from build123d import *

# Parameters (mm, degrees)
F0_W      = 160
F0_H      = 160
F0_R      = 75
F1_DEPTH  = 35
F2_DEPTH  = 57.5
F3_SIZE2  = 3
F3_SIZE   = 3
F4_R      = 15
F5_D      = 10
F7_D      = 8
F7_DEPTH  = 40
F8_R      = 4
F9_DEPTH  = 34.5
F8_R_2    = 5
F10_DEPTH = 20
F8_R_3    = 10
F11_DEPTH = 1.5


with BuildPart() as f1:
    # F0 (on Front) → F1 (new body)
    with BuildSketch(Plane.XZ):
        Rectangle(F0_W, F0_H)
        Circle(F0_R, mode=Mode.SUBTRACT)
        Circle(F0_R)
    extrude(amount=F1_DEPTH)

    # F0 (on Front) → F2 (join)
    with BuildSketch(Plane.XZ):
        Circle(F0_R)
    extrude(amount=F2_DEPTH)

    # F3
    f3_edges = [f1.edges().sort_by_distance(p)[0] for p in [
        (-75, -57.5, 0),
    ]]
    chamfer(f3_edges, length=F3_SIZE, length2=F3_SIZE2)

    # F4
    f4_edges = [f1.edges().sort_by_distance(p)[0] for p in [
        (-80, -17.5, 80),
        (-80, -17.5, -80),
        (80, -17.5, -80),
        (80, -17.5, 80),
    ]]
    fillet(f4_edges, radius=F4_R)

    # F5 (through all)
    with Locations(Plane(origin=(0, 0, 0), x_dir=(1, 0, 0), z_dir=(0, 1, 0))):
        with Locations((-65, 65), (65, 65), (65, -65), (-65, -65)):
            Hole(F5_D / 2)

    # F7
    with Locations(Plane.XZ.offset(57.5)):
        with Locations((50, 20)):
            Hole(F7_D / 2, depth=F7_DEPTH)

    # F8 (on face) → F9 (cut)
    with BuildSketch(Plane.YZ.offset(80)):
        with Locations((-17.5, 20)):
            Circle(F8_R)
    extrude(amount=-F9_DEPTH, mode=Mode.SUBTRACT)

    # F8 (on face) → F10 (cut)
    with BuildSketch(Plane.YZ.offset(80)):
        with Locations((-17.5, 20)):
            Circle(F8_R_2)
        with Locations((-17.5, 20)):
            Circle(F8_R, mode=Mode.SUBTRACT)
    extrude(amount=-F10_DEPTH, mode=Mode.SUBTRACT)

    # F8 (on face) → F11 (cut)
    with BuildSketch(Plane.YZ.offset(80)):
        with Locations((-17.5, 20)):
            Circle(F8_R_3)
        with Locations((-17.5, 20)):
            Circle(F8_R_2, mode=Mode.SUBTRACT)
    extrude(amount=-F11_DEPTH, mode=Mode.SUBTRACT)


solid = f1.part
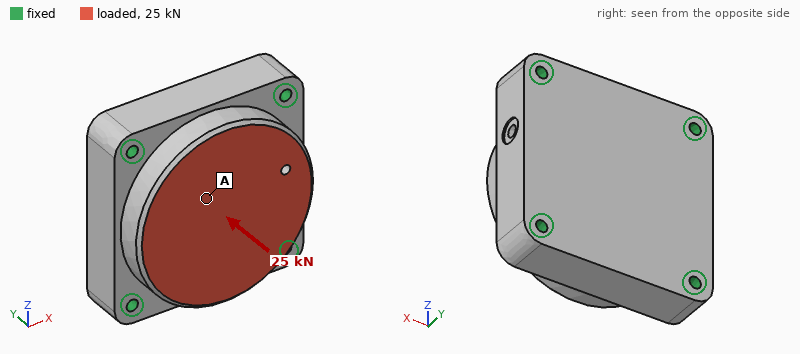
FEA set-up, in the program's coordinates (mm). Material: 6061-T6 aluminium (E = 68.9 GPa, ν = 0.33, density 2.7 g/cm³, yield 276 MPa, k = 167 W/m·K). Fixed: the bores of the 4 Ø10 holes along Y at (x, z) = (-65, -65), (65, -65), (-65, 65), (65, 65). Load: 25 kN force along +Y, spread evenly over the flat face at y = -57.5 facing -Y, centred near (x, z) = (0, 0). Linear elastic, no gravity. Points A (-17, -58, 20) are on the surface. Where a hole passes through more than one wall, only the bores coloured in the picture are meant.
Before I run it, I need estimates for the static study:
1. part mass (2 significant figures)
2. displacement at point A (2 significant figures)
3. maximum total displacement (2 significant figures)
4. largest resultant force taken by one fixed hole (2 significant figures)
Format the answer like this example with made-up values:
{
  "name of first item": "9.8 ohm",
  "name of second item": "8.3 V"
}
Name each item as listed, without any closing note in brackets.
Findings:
{
  "part mass": "3.4 kg",
  "displacement at point A": "9.3 µm",
  "maximum total displacement": "9.8 µm",
  "largest resultant force taken by one fixed hole": "6.6 kN"
}
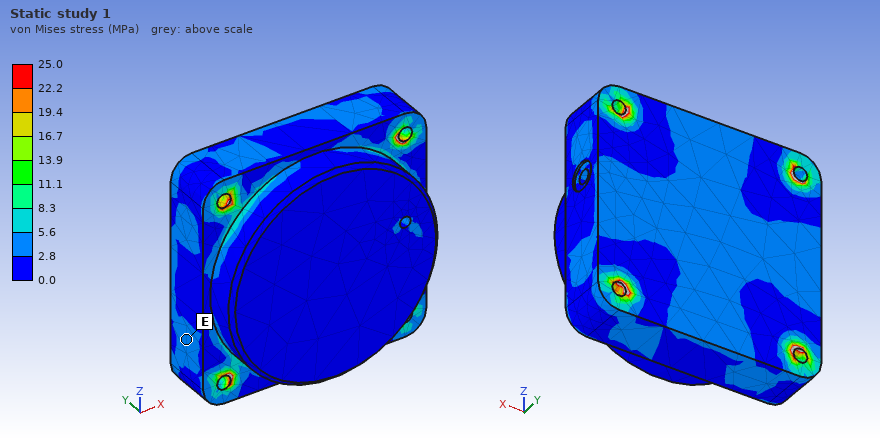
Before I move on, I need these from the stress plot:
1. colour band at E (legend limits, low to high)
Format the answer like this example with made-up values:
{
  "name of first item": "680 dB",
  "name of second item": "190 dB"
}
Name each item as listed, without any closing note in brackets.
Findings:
{
  "colour band at E": "2.8 to 5.6 MPa"
}
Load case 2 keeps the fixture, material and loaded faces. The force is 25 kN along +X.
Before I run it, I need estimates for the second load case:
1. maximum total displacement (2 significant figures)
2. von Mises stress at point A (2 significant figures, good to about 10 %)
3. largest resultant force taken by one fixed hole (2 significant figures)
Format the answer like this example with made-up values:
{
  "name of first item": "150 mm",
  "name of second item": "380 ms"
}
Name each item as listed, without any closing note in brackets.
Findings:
{
  "maximum total displacement": "10 µm",
  "von Mises stress at point A": "3.1 MPa",
  "largest resultant force taken by one fixed hole": "7.8 kN"
}
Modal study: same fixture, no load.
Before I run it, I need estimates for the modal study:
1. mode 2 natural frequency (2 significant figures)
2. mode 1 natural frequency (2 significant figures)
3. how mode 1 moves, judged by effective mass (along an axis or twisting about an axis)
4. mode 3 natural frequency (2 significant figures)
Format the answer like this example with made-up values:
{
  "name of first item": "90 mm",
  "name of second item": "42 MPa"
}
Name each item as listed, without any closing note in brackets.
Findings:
{
  "mode 2 natural frequency": "7200 Hz",
  "mode 1 natural frequency": "5200 Hz",
  "how mode 1 moves, judged by effective mass": "along Y",
  "mode 3 natural frequency": "7200 Hz"
}
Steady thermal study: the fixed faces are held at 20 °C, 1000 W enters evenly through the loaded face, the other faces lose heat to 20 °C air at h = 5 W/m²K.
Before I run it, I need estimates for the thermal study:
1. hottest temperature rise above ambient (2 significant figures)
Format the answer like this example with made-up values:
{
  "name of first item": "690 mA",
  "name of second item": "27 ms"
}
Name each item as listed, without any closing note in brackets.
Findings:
{
  "hottest temperature rise above ambient": "42 K"
}
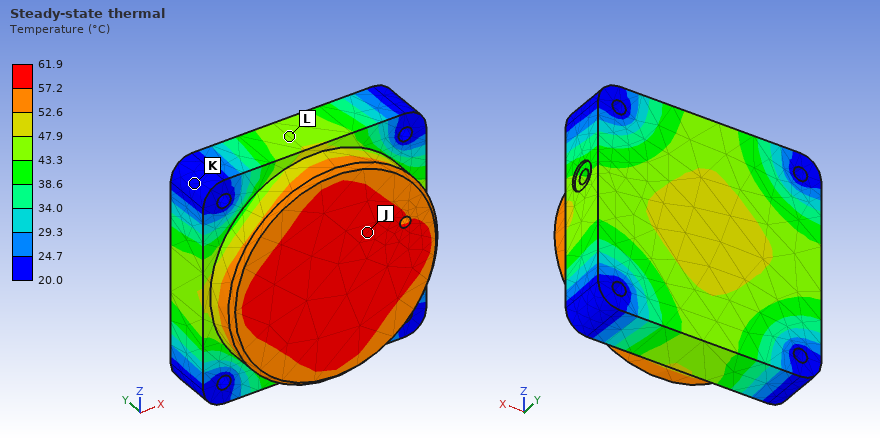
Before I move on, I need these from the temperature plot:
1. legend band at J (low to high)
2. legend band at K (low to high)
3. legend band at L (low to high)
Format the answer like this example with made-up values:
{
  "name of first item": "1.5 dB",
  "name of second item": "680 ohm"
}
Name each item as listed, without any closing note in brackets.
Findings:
{
  "legend band at J": "57.2 to 61.9 °C",
  "legend band at K": "20.0 to 24.7 °C",
  "legend band at L": "43.3 to 47.9 °C"
}
